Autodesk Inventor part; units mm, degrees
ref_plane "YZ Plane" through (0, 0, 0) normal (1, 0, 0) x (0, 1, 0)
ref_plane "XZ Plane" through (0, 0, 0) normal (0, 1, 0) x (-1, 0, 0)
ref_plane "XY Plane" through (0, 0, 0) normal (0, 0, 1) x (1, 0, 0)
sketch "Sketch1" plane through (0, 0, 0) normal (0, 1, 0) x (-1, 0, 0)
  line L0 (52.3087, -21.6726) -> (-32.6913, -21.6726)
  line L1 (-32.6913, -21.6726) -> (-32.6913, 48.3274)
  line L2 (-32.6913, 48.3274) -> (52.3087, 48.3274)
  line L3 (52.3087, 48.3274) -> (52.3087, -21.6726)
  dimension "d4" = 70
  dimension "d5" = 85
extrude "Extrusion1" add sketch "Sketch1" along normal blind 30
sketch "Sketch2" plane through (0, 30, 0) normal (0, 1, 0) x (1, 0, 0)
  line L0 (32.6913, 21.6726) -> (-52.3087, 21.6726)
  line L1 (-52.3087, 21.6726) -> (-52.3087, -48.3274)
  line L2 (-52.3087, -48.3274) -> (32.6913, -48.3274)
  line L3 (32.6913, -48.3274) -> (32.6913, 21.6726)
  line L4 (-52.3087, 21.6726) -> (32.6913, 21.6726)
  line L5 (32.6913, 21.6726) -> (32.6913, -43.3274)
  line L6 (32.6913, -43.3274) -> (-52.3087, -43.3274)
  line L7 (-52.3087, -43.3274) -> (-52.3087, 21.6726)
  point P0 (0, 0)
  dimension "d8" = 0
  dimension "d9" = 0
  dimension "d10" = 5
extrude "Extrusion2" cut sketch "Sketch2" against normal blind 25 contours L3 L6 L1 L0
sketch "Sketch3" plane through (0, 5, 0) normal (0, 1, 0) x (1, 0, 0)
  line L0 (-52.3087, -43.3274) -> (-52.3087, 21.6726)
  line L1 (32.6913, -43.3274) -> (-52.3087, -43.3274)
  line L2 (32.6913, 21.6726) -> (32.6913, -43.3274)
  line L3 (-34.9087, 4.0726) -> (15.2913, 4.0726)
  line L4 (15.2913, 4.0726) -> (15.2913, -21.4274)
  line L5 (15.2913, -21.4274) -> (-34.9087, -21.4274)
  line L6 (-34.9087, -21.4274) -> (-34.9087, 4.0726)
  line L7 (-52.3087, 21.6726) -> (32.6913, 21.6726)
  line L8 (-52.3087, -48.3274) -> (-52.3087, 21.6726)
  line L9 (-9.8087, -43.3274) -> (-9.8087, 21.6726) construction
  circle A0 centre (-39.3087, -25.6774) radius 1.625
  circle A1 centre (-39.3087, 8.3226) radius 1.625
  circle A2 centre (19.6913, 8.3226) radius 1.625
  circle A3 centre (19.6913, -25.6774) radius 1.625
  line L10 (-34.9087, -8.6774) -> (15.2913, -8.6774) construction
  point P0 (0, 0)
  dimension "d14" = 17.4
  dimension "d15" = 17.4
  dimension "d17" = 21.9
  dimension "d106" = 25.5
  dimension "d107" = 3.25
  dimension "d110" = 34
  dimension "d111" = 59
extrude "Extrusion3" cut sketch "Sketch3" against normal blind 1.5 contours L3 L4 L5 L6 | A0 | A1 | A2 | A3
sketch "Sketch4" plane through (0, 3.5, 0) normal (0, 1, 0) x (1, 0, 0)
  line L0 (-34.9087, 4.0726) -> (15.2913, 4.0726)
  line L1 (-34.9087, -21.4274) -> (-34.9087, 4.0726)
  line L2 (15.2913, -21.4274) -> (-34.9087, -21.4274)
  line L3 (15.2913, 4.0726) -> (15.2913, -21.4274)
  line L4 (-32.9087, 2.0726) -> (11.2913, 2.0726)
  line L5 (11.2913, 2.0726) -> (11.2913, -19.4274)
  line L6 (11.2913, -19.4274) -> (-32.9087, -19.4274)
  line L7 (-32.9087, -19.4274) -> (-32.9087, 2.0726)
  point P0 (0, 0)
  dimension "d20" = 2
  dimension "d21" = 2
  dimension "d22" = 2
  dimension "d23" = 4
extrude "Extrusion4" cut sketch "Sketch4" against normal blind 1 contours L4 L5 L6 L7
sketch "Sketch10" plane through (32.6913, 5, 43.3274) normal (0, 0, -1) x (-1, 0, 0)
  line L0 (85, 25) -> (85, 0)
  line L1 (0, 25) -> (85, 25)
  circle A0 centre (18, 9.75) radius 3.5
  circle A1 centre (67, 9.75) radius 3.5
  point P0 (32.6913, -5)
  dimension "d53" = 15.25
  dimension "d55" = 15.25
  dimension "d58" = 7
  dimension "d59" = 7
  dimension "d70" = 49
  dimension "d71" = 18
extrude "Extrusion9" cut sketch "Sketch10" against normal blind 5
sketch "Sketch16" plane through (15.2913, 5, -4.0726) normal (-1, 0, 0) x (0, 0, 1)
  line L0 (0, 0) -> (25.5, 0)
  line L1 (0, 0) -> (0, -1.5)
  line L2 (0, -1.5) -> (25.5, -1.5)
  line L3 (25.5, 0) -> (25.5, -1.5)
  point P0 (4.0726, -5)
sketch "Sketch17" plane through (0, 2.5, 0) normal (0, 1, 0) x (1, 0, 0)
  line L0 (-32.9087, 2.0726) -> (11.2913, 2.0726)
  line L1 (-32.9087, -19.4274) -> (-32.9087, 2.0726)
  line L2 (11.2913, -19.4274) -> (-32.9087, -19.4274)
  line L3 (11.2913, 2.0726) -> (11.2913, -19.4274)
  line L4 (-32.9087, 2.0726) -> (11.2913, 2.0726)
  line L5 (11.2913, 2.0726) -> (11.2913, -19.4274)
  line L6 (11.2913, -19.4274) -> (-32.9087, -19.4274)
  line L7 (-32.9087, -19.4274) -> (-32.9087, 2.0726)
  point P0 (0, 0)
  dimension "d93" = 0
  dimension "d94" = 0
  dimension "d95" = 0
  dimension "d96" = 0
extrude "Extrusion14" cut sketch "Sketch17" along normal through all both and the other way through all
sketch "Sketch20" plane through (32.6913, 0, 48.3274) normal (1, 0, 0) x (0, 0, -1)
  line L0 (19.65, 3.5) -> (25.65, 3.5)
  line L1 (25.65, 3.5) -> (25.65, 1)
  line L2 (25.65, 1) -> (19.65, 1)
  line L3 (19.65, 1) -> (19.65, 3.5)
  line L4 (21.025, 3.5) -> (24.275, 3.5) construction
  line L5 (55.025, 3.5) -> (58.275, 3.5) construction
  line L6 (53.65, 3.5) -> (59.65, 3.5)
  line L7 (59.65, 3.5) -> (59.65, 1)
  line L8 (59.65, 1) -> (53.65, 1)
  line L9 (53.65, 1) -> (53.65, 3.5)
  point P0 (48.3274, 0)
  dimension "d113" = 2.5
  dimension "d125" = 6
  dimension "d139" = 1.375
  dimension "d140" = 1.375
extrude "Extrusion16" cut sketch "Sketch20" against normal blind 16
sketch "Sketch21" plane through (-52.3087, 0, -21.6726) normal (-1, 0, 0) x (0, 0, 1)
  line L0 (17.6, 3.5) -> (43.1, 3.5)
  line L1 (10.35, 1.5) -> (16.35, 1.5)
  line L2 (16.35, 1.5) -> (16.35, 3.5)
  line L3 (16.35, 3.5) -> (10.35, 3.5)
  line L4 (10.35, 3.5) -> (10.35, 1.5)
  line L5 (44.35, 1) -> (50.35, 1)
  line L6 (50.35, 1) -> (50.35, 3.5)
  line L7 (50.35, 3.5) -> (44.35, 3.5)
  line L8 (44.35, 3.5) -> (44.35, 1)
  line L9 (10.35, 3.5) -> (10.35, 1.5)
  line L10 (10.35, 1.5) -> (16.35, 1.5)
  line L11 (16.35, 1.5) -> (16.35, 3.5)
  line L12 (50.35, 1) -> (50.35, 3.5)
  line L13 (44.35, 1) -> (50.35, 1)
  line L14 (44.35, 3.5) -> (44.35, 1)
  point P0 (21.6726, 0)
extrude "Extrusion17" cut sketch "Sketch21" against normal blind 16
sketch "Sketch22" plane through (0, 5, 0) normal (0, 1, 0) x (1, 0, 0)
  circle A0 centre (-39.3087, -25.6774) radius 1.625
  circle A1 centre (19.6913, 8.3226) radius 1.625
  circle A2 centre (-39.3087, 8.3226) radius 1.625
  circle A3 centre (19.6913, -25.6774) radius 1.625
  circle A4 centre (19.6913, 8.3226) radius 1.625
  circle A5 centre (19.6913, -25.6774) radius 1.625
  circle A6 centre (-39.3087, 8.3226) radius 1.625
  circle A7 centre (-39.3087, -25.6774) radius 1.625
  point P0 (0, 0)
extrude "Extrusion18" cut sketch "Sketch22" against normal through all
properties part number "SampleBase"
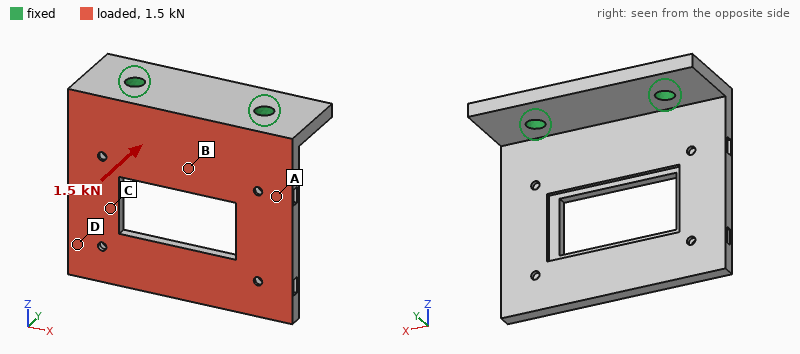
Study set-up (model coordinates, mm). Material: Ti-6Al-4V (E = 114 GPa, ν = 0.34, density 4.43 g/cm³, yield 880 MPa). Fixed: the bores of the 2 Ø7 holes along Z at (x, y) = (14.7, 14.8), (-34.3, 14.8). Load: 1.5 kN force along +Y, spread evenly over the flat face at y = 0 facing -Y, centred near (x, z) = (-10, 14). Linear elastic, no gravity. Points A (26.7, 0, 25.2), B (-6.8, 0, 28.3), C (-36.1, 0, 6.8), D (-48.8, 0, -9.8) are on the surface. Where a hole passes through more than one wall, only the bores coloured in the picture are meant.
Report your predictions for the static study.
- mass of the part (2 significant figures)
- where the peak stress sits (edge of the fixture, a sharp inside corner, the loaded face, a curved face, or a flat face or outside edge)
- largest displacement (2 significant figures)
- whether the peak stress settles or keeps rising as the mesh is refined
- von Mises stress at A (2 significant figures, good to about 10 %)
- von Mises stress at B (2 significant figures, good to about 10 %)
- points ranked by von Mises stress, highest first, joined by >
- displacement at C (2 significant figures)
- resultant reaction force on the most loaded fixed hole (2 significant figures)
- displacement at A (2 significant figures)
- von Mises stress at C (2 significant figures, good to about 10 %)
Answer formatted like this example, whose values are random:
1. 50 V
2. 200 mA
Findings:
1. 150 g
2. edge of the fixture
3. 1.1 mm
4. keeps rising
5. 120 MPa
6. 41 MPa
7. A > C > B > D
8. 0.51 mm
9. 760 N
10. 0.21 mm
11. 68 MPa
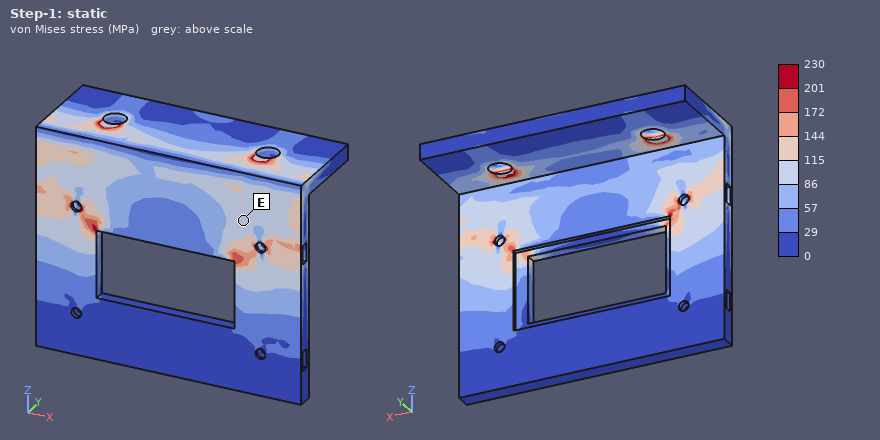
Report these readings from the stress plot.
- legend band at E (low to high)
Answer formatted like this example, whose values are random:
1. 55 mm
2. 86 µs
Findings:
1. 86 to 115 MPa
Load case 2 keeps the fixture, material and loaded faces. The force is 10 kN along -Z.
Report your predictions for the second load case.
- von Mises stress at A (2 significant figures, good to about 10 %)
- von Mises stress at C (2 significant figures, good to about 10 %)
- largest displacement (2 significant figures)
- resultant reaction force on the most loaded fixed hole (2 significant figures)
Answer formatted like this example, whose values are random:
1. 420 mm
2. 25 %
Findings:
1. 130 MPa
2. 100 MPa
3. 1.2 mm
4. 5.0 kN
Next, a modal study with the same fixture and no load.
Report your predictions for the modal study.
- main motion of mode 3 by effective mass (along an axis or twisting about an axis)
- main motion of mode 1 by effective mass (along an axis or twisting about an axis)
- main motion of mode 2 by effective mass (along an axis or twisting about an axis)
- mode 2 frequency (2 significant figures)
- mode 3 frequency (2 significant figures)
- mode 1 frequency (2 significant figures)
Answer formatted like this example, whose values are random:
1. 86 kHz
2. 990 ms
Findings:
1. along X
2. along Y
3. twisting about Z
4. 1400 Hz
5. 3200 Hz
6. 680 Hz
